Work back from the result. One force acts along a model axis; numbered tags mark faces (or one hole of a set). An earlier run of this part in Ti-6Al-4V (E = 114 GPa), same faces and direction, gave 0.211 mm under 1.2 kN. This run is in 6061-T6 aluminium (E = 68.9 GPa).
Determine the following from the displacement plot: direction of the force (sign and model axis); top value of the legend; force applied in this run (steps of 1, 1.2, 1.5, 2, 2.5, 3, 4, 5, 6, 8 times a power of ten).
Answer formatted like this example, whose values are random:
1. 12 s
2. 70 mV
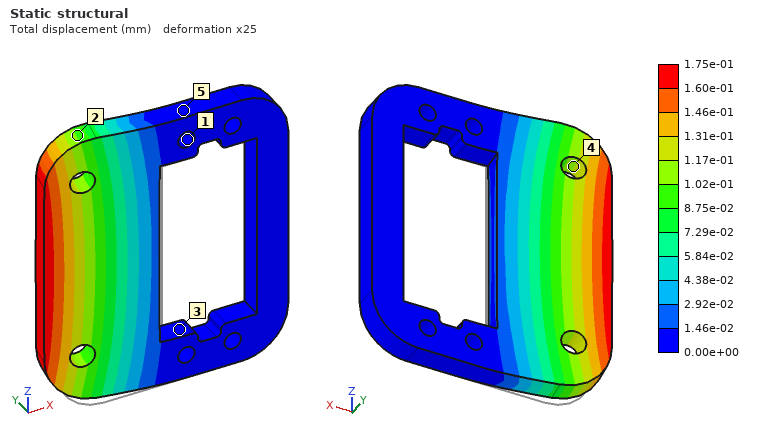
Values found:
1. +Y
2. 1.75e-01 mm
3. 600 N
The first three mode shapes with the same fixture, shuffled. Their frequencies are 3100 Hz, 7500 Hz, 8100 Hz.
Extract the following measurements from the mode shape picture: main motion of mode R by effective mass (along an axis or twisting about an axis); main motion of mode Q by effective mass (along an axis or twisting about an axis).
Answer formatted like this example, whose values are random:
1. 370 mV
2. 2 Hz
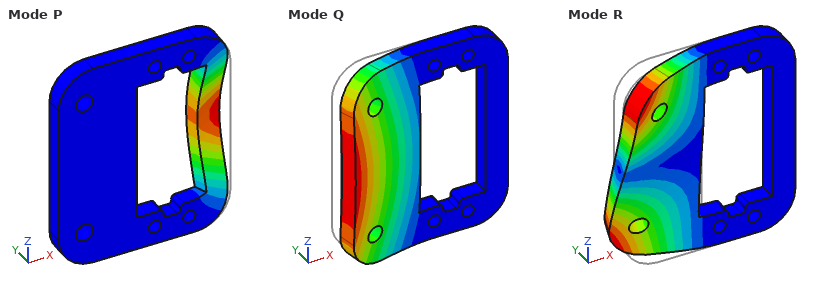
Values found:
1. twisting about X
2. along Y
